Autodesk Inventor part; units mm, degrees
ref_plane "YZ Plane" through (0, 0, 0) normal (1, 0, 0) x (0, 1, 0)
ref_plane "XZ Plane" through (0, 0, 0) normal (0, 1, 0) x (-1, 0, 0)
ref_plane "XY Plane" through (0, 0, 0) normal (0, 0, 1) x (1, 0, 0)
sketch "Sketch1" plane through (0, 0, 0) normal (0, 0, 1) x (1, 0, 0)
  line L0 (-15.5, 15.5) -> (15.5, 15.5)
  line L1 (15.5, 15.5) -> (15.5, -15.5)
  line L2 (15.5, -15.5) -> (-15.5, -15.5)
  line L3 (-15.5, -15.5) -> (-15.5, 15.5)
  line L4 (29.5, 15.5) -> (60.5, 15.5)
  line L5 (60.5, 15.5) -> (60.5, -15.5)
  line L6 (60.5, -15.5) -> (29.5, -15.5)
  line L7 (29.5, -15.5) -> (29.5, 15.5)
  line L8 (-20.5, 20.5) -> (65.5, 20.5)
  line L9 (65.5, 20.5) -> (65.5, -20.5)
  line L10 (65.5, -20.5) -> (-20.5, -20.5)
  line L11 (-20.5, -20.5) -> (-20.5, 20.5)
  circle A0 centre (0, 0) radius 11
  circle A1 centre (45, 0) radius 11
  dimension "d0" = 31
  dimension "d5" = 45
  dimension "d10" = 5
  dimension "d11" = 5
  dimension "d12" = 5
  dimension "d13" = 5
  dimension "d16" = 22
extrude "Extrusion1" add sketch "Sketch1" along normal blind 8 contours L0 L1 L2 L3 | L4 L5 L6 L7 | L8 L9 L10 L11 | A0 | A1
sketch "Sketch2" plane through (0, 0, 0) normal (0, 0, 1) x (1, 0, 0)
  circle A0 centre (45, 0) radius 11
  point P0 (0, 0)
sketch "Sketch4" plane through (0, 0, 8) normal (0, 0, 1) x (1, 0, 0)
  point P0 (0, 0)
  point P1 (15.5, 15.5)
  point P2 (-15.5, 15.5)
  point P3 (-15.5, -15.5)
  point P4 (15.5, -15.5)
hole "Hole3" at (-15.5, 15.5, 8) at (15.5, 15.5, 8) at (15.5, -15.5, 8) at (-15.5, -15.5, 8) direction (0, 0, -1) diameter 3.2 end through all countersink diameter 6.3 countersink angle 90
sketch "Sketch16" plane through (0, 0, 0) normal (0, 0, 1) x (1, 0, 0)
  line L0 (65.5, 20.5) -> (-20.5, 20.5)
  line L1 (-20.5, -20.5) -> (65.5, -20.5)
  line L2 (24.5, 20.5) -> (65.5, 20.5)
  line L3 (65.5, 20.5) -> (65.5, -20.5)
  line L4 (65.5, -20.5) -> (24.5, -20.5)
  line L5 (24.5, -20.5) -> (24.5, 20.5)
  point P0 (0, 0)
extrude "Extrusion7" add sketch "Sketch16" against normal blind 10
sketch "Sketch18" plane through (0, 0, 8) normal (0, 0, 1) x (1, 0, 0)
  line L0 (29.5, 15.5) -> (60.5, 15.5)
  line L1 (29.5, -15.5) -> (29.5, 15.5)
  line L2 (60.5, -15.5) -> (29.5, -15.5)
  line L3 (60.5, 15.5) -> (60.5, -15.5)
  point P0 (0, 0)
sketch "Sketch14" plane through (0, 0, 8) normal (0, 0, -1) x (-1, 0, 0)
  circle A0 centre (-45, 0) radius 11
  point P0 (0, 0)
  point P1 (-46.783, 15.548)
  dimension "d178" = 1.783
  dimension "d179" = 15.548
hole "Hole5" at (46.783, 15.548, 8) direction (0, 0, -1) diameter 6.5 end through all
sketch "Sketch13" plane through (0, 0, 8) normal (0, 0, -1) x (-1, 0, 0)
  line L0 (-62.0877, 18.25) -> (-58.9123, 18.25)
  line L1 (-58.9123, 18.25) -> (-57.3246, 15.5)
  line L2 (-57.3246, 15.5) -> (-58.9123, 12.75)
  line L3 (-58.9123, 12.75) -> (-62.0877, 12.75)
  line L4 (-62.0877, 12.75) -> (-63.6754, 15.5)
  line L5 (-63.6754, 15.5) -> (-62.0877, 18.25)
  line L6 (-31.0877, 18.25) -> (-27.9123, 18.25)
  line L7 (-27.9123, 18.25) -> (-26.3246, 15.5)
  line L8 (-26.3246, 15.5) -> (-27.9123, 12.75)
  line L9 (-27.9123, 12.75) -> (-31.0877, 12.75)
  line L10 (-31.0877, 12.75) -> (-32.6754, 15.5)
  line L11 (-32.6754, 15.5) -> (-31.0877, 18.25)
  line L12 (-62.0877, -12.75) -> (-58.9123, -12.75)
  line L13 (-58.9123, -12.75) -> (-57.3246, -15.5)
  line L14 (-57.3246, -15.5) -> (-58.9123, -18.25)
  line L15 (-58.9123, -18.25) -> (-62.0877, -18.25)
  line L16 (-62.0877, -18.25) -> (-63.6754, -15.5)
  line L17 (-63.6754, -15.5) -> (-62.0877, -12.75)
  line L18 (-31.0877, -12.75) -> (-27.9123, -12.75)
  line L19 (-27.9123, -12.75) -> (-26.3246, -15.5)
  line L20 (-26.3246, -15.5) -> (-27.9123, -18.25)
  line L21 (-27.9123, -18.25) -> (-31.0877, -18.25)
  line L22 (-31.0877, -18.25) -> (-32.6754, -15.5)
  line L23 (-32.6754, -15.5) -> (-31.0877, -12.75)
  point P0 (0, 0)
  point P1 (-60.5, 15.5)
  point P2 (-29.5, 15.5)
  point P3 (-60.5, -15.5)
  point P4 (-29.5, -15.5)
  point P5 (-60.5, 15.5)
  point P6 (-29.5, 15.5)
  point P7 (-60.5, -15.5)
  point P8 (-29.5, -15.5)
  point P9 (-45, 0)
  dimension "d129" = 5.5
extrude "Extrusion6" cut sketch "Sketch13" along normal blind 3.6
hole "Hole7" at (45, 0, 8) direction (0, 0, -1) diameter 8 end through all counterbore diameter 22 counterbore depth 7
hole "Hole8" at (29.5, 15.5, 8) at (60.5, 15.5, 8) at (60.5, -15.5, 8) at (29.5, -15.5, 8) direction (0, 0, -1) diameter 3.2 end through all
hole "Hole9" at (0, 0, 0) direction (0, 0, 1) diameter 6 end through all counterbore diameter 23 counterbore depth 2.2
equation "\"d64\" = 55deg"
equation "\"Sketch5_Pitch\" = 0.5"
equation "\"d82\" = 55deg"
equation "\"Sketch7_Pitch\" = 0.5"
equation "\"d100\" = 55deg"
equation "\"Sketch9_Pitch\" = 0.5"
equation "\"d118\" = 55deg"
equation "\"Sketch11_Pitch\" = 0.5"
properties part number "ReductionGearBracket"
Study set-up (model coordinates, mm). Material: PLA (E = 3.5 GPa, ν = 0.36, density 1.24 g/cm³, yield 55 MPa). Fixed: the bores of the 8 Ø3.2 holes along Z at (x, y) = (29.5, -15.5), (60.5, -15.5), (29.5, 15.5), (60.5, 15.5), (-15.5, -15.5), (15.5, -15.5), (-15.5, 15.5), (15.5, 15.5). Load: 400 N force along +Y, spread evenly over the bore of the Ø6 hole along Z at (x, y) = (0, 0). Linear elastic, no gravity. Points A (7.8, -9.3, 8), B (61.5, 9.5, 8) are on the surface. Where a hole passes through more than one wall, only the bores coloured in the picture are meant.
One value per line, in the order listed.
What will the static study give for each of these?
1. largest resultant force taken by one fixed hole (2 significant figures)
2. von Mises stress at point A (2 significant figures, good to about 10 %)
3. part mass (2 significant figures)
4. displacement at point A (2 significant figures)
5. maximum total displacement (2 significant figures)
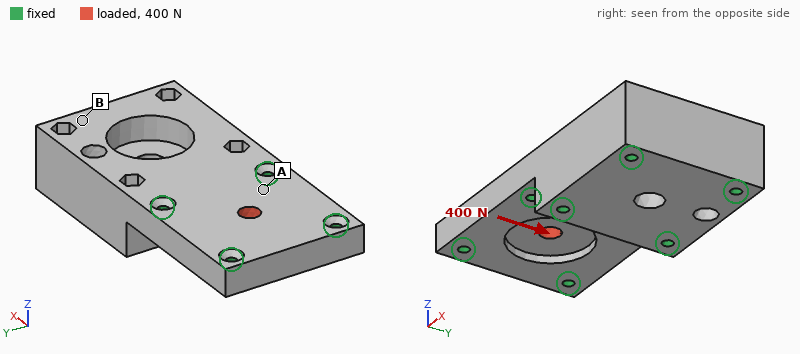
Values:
110 N
1.7 MPa
48 g
6.1 µm
14 µm
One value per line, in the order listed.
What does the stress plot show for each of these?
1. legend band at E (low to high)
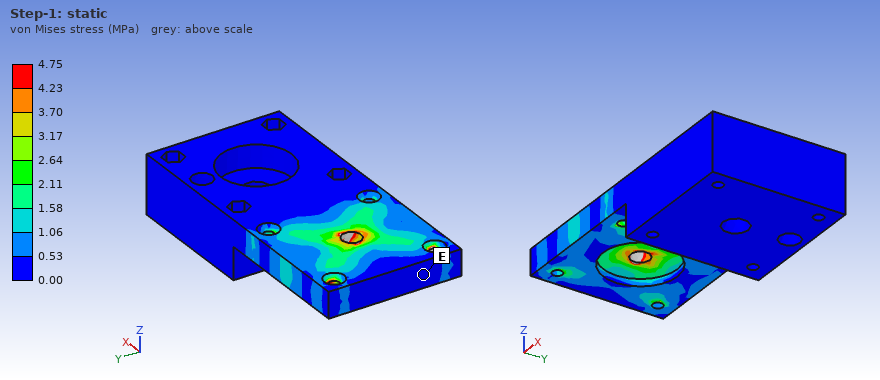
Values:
0.00 to 0.53 MPa
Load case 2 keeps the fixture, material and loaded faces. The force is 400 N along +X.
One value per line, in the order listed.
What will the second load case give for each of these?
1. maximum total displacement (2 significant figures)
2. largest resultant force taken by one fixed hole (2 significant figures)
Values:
14 µm
93 N
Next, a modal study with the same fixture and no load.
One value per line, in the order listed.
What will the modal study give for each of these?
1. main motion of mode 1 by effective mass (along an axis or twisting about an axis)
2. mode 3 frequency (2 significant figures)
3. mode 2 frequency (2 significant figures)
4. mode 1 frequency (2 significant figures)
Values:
along Z
10 kHz
10 kHz
7400 Hz
